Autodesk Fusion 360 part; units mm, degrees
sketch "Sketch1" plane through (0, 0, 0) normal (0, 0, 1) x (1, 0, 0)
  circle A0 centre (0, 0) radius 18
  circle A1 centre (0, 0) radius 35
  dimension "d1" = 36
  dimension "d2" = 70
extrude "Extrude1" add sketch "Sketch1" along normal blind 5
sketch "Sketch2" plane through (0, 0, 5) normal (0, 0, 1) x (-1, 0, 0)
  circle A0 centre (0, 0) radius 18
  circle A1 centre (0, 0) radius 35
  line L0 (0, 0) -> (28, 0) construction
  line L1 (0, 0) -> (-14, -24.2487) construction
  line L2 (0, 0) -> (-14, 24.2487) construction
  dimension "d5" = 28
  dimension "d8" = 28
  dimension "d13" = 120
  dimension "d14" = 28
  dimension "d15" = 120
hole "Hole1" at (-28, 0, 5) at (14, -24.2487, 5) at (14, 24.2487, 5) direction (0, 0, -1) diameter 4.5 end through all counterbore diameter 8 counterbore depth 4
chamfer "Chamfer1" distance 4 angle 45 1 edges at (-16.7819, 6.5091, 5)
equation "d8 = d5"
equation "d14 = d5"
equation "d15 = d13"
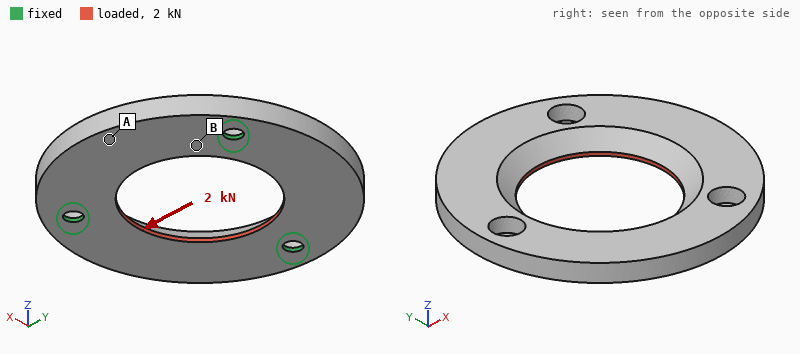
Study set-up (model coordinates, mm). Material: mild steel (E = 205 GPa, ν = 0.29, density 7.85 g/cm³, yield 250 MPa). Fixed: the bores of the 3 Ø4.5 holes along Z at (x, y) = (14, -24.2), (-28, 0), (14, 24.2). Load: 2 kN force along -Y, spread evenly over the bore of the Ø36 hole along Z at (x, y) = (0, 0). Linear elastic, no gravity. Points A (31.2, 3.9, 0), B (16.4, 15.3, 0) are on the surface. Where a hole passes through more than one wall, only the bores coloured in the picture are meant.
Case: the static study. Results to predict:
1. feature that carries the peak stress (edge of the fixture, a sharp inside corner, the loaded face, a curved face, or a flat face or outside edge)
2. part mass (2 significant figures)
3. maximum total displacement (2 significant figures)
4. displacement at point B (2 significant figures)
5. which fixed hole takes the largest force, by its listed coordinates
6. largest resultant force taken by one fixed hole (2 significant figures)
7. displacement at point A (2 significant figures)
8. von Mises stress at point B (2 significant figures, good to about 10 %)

edge of the fixture
98 g
3.9 µm
1.2 µm
(-28, 0)
800 N
1.5 µm
16 MPa
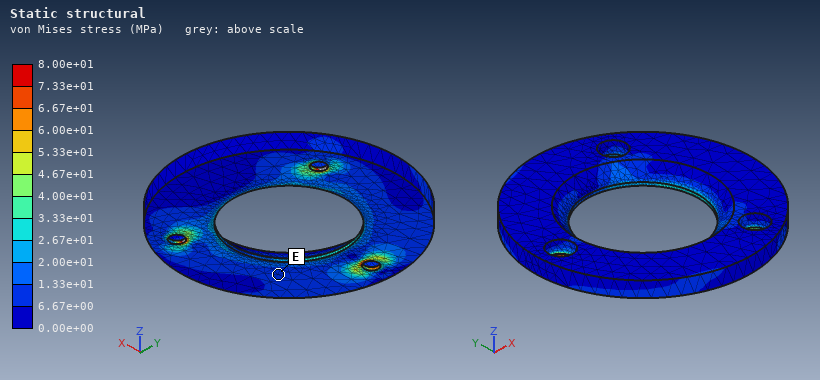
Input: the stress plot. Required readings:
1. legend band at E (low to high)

6.67e+00 to 1.33e+01 MPa
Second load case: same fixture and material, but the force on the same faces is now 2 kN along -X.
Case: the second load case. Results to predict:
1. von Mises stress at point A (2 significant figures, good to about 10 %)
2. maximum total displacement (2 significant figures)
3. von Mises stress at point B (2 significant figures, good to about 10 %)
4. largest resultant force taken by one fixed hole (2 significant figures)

7.3 MPa
4.2 µm
13 MPa
740 N
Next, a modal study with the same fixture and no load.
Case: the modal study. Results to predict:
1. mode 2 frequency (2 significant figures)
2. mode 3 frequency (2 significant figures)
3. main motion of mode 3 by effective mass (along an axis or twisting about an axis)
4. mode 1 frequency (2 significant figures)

3400 Hz
5500 Hz
along Z
3400 Hz
